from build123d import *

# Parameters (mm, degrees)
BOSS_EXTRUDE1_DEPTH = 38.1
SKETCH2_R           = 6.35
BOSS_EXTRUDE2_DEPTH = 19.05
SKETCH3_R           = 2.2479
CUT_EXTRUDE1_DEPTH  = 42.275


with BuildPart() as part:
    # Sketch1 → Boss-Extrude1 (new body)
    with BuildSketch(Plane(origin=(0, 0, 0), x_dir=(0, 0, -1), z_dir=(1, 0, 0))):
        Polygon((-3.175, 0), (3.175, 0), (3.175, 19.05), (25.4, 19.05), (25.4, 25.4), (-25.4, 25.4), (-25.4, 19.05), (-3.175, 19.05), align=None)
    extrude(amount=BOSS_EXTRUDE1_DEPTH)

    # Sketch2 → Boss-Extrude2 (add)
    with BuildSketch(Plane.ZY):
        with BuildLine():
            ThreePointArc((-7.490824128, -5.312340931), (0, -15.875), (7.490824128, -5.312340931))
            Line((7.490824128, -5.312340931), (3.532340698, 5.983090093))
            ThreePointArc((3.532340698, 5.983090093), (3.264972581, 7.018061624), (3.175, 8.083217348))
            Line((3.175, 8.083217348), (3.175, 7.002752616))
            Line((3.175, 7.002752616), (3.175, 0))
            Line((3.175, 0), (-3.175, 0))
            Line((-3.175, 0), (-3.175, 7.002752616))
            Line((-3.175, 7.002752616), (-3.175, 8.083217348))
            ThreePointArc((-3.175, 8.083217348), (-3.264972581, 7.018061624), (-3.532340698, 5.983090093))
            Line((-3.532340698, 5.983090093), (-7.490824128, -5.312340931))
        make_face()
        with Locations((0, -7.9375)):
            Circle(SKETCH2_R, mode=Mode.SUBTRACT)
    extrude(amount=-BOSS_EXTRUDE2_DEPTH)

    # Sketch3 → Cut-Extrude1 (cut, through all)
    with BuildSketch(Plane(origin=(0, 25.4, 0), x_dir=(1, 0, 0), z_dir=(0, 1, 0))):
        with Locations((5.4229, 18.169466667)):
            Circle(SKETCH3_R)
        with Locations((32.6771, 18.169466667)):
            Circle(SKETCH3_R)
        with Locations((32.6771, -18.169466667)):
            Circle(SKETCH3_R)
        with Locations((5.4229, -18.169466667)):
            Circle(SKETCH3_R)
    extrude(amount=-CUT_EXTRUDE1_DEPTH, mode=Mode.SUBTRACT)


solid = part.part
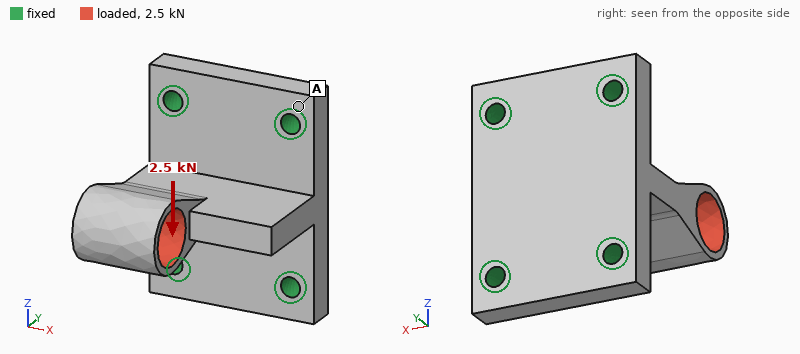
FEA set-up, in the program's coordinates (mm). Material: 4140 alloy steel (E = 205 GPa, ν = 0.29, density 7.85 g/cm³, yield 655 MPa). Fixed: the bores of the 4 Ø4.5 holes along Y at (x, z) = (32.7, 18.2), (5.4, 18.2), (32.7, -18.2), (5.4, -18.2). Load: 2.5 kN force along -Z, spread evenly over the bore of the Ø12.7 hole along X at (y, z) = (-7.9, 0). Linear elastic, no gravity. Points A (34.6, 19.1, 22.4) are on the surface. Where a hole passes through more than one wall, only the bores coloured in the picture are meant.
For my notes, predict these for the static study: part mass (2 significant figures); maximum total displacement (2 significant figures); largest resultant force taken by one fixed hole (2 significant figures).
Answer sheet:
140 g
0.30 mm
1.9 kN
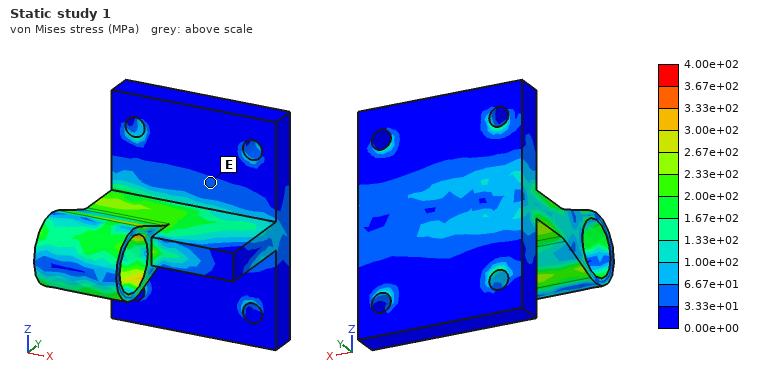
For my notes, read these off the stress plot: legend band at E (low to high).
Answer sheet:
3.33e+01 to 6.67e+01 MPa
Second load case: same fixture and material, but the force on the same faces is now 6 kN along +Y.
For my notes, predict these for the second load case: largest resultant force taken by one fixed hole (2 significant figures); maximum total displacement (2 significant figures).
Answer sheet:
2.5 kN
59 µm
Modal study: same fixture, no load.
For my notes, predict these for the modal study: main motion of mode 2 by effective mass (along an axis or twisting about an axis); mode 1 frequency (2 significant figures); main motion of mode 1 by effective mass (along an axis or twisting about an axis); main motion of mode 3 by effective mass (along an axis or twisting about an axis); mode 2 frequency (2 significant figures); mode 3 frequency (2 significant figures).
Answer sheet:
along X
4500 Hz
along Z
along Y
8500 Hz
13 kHz
